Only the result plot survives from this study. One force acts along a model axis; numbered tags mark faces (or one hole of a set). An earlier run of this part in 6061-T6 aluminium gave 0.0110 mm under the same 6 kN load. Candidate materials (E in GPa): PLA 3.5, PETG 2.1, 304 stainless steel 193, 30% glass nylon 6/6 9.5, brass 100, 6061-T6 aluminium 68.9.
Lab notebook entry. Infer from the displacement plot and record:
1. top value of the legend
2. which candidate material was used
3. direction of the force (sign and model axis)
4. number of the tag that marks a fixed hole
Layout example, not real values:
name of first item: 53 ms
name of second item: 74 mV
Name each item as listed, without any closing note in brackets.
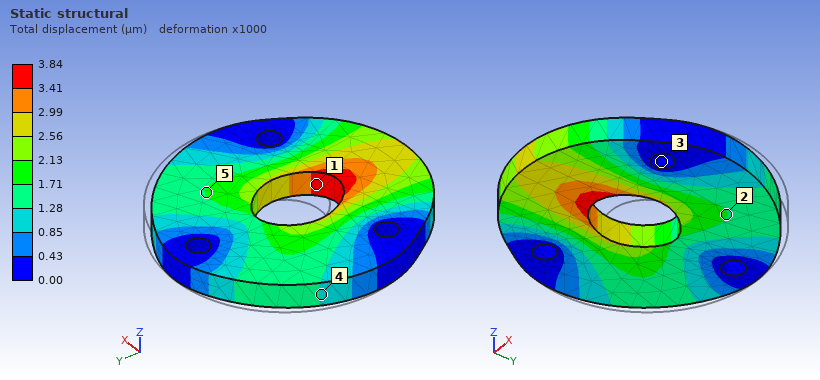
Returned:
top value of the legend: 3.84 µm
which candidate material was used: 304 stainless steel
direction of the force: -Y
number of the tag that marks a fixed hole: 3
